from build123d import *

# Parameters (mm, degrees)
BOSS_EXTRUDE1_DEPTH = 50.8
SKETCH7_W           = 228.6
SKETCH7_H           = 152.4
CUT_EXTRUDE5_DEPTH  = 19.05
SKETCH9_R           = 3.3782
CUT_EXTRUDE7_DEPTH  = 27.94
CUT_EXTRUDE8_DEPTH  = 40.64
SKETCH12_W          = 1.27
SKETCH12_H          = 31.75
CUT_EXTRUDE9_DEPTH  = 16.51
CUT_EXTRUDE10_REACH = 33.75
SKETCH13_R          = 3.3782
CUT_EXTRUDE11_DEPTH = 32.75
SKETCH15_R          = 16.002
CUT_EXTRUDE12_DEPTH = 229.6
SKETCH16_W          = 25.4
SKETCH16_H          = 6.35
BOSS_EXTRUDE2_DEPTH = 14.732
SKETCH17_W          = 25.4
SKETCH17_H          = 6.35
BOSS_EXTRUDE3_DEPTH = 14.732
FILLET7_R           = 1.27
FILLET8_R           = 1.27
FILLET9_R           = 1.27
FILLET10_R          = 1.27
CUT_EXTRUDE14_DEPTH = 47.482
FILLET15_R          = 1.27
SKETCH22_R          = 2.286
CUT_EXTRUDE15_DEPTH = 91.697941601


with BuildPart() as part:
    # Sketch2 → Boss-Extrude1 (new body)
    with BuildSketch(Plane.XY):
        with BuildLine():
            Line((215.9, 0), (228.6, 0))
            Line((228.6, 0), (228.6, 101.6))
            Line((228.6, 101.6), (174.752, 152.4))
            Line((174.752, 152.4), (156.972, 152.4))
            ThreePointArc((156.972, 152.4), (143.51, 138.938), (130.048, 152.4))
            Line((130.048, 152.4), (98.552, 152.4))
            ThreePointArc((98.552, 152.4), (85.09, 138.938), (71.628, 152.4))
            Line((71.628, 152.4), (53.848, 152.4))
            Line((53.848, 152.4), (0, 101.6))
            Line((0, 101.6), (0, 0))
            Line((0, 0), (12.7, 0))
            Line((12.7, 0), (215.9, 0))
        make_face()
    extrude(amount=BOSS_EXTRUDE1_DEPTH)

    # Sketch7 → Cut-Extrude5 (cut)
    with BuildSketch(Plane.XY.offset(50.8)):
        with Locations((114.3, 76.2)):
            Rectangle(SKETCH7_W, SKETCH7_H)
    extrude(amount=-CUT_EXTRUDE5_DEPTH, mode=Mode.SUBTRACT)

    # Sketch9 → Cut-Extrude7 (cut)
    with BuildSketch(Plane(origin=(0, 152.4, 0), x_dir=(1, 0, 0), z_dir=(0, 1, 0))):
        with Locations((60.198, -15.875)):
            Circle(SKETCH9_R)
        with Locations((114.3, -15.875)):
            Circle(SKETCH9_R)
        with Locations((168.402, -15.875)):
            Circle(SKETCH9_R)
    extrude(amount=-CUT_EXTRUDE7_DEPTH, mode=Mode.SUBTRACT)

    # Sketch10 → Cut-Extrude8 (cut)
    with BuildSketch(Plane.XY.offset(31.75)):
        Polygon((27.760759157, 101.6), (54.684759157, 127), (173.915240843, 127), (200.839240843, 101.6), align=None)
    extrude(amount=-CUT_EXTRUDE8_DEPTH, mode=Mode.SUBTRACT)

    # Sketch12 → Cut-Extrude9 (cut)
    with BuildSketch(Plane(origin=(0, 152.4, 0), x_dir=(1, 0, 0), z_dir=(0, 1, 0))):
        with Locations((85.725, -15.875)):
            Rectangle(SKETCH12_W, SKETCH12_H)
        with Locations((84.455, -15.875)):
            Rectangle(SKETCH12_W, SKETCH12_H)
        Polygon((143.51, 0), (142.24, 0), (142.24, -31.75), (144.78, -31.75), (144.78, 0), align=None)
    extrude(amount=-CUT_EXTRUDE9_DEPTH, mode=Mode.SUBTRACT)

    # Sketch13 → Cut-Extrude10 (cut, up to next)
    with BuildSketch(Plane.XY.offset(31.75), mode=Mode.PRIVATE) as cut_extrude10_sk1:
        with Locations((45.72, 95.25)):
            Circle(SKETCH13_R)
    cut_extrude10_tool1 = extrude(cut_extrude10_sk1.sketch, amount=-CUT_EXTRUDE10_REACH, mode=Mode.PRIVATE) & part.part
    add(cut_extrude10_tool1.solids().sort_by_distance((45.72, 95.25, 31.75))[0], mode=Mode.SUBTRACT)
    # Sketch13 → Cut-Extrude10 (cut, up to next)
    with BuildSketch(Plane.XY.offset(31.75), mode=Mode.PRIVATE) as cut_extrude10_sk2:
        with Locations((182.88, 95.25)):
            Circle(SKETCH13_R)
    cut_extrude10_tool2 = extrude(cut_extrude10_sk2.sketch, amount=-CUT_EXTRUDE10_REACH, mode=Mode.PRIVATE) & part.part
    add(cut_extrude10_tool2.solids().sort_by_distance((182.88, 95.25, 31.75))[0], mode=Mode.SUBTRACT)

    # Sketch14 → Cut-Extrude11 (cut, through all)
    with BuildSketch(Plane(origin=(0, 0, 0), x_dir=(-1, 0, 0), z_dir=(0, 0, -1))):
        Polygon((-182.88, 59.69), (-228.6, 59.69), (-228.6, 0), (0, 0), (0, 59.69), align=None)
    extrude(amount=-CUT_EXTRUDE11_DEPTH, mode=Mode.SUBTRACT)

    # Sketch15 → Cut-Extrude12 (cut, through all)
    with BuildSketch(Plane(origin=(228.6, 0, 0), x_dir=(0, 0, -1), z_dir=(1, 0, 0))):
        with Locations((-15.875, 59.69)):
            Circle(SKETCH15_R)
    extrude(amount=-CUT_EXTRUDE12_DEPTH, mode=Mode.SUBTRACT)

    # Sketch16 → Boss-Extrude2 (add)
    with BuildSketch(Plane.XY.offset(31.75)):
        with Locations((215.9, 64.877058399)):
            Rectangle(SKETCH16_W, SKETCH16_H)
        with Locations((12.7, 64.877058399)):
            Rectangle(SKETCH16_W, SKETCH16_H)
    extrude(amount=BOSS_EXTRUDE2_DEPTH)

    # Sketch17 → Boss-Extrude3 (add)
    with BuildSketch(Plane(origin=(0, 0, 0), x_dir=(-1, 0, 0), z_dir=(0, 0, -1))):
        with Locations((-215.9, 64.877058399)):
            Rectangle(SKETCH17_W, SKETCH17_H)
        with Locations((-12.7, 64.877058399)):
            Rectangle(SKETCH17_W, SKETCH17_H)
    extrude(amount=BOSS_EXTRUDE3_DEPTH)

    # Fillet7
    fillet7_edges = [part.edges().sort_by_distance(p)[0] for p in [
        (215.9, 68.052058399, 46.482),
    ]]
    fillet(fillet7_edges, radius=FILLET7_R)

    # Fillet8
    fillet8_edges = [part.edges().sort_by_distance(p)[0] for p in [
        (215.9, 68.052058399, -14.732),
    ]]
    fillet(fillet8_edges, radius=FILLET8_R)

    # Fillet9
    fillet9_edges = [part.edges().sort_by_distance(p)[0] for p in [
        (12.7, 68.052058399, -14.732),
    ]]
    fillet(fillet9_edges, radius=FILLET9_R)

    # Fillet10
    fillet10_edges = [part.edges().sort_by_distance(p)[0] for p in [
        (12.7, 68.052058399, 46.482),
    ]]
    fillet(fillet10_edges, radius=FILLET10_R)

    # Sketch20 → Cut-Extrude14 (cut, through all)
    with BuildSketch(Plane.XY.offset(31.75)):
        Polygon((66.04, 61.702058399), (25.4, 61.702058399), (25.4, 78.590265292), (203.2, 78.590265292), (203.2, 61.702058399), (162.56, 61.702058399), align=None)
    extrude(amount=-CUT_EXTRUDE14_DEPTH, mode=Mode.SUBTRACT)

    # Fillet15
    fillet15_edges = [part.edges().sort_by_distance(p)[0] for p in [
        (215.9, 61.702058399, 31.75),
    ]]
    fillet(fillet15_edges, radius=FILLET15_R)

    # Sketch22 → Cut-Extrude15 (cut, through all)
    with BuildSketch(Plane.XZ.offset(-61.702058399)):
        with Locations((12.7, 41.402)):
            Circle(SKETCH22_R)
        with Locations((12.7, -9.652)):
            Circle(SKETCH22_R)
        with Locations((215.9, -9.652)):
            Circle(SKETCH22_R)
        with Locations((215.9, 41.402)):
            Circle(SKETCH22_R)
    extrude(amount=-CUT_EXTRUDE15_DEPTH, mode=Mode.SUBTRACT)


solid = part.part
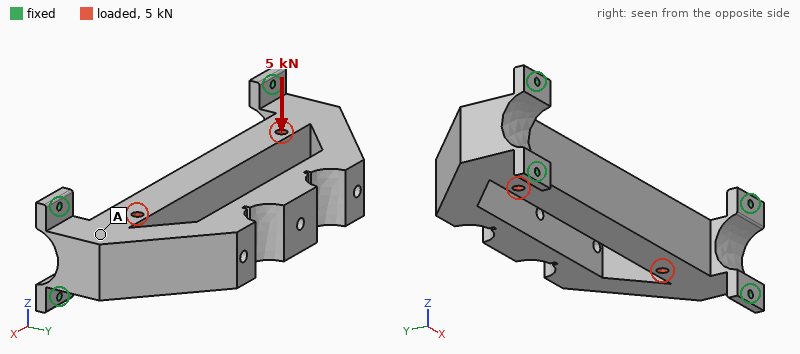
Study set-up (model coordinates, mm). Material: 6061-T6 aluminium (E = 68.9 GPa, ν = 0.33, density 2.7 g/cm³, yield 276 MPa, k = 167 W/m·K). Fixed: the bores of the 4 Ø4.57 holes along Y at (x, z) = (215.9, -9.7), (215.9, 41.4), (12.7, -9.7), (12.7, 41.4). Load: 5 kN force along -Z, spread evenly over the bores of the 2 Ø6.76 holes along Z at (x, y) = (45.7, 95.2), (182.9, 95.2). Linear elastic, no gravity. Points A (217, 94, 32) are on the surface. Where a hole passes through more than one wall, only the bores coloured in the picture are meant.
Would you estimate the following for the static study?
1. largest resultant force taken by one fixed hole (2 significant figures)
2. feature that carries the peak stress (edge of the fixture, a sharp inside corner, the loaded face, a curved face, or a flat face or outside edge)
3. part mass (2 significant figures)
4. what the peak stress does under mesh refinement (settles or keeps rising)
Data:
2.6 kN
edge of the fixture
880 g
keeps rising
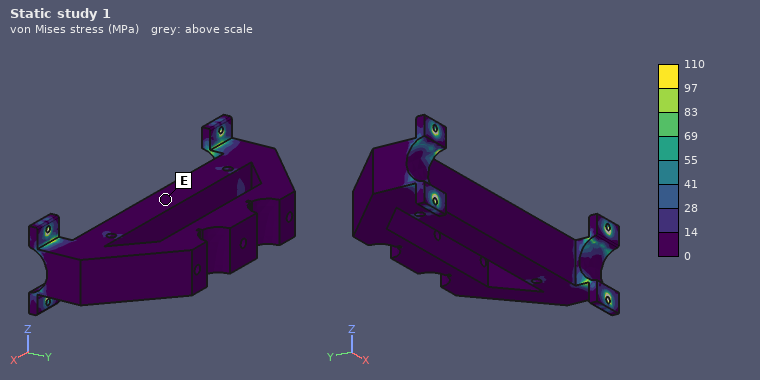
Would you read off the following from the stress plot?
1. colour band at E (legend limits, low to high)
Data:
0 to 14 MPa
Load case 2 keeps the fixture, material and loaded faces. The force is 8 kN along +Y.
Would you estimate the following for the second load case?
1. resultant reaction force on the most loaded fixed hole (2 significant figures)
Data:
2.5 kN
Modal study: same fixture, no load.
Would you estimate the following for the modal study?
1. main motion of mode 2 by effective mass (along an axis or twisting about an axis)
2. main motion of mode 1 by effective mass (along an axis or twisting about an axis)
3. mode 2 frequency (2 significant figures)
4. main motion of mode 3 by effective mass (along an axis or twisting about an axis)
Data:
along X
along Z
1500 Hz
along Y
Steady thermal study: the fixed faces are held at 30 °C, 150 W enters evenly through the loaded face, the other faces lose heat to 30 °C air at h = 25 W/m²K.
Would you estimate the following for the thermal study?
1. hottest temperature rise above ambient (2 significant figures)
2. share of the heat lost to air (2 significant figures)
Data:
50 K
33 %
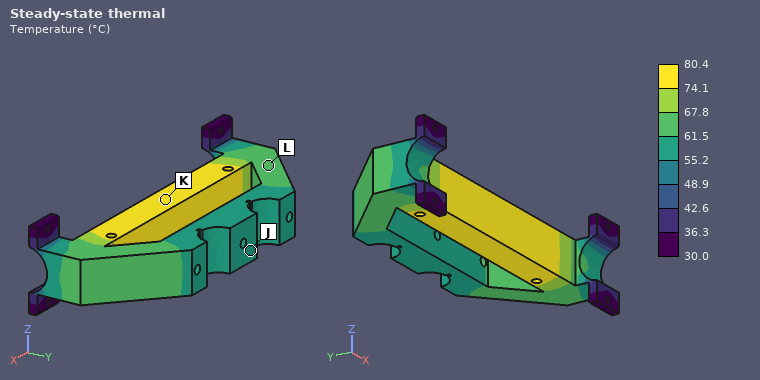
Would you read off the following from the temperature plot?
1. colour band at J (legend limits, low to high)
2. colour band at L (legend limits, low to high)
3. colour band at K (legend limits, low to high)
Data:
55.2 to 61.5 °C
61.5 to 67.8 °C
74.1 to 80.4 °C
